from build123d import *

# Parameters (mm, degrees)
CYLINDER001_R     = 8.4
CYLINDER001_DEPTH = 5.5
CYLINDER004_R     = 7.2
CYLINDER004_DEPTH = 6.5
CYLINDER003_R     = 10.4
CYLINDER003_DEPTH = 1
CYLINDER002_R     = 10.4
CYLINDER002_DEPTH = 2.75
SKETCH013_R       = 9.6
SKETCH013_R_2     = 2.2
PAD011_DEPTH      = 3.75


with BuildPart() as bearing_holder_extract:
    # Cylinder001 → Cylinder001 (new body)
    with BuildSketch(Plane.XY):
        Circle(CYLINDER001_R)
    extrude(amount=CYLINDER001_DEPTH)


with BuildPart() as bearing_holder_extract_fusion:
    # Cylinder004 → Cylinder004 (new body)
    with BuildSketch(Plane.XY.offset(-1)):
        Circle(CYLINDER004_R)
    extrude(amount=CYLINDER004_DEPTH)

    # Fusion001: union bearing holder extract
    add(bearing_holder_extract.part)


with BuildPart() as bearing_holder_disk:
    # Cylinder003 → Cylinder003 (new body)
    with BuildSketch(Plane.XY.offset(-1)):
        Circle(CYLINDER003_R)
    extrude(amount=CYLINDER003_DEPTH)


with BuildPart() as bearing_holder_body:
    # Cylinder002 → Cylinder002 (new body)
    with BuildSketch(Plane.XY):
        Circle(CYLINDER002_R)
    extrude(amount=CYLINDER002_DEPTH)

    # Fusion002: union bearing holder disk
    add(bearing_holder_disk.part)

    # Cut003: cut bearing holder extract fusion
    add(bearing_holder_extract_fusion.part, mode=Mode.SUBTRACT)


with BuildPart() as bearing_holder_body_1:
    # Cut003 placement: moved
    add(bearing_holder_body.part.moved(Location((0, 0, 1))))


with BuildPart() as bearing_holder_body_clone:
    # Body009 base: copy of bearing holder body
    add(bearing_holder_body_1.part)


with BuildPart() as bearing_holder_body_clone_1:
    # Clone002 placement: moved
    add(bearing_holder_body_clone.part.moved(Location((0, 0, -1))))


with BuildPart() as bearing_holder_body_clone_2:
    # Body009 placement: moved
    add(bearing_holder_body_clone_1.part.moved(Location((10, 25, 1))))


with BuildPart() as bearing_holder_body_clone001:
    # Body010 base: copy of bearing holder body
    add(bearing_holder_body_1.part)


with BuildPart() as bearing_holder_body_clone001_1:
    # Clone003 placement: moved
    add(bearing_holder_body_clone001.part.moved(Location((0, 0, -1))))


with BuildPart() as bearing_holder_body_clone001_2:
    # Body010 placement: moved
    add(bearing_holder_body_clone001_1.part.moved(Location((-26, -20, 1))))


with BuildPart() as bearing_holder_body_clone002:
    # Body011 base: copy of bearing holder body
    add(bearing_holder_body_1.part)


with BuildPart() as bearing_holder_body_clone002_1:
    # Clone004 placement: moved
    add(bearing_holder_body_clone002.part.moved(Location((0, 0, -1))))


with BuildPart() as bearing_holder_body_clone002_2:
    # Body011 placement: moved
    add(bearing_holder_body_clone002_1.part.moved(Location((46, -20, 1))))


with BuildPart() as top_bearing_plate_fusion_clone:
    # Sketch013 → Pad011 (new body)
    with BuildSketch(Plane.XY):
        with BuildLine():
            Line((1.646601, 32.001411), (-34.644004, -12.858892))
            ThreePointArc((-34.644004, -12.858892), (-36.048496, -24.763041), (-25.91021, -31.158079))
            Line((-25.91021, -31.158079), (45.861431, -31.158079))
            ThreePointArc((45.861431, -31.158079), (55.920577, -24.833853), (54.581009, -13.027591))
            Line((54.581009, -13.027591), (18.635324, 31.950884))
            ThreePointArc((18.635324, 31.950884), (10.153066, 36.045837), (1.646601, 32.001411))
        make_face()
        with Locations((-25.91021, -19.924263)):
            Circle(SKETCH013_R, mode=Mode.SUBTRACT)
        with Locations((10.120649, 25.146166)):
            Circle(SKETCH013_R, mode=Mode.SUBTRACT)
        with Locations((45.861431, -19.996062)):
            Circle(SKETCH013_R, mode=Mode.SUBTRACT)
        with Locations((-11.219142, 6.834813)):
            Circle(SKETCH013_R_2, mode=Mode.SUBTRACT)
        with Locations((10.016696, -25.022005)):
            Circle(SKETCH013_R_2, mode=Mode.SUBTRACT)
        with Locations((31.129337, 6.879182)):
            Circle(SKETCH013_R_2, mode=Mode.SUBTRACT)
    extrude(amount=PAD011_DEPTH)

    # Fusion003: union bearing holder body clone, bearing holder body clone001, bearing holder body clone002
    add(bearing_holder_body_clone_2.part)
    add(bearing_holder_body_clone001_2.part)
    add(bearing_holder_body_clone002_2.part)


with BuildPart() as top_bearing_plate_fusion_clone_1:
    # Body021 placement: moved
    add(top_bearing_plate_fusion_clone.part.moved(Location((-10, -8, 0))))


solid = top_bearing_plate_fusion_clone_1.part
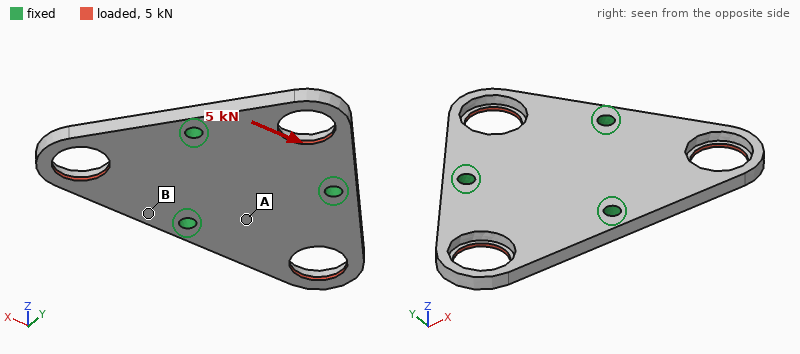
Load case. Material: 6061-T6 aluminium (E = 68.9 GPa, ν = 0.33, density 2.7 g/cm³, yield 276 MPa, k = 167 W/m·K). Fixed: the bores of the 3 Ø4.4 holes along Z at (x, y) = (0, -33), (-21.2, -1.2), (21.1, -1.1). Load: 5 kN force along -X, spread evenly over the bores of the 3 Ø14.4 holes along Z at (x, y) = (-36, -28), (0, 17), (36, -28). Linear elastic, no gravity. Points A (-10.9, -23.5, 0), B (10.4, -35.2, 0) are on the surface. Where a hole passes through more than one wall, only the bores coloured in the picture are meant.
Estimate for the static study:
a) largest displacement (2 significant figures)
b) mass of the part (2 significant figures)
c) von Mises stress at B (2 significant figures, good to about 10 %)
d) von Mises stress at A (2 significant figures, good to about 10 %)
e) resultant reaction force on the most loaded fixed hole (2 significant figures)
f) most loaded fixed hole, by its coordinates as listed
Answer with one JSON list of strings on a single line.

["0.17 mm", "35 g", "42 MPa", "19 MPa", "2.5 kN", "(0, -33)"]
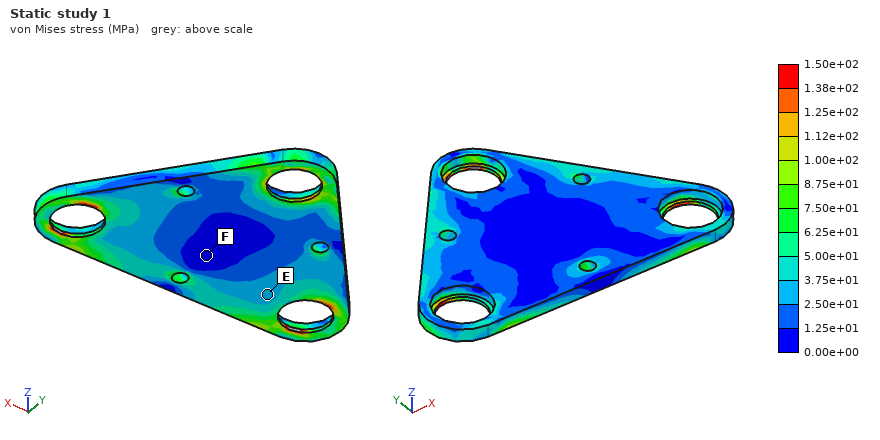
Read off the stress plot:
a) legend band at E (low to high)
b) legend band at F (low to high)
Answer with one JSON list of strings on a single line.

["2.50e+01 to 3.75e+01 MPa", "0.00e+00 to 1.25e+01 MPa"]
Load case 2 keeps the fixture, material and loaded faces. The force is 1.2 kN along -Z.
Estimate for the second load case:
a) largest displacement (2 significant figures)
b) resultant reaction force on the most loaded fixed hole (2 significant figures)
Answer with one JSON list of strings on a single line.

["0.48 mm", "450 N"]
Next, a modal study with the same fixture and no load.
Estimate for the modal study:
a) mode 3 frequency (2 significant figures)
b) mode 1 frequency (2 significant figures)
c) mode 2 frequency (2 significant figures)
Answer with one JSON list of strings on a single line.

["5200 Hz", "3400 Hz", "3500 Hz"]
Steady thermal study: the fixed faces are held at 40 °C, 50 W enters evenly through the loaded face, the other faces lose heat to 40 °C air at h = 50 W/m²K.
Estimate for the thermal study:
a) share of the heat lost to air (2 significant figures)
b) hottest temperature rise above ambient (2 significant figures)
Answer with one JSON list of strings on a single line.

["11 %", "43 K"]
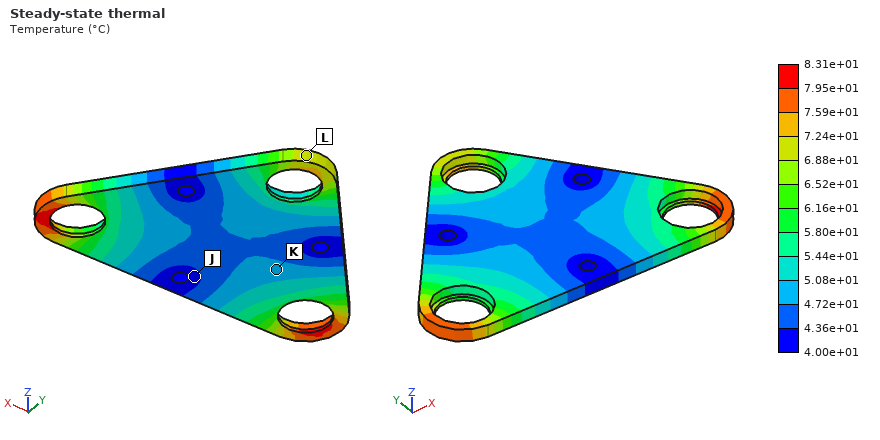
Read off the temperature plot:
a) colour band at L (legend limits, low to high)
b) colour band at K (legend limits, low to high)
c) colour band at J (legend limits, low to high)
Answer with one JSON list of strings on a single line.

["6.88e+01 to 7.24e+01 °C", "4.72e+01 to 5.08e+01 °C", "4.00e+01 to 4.36e+01 °C"]
